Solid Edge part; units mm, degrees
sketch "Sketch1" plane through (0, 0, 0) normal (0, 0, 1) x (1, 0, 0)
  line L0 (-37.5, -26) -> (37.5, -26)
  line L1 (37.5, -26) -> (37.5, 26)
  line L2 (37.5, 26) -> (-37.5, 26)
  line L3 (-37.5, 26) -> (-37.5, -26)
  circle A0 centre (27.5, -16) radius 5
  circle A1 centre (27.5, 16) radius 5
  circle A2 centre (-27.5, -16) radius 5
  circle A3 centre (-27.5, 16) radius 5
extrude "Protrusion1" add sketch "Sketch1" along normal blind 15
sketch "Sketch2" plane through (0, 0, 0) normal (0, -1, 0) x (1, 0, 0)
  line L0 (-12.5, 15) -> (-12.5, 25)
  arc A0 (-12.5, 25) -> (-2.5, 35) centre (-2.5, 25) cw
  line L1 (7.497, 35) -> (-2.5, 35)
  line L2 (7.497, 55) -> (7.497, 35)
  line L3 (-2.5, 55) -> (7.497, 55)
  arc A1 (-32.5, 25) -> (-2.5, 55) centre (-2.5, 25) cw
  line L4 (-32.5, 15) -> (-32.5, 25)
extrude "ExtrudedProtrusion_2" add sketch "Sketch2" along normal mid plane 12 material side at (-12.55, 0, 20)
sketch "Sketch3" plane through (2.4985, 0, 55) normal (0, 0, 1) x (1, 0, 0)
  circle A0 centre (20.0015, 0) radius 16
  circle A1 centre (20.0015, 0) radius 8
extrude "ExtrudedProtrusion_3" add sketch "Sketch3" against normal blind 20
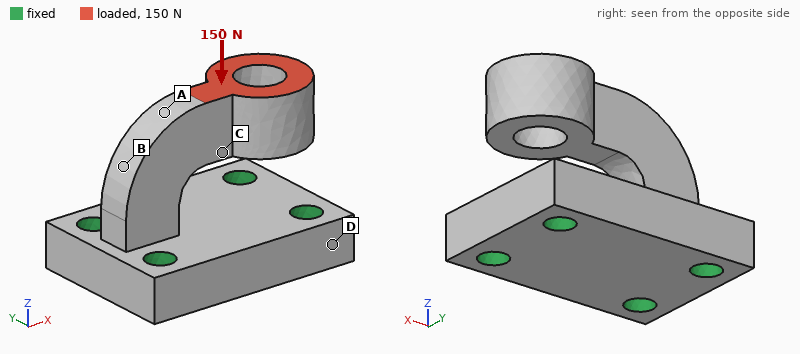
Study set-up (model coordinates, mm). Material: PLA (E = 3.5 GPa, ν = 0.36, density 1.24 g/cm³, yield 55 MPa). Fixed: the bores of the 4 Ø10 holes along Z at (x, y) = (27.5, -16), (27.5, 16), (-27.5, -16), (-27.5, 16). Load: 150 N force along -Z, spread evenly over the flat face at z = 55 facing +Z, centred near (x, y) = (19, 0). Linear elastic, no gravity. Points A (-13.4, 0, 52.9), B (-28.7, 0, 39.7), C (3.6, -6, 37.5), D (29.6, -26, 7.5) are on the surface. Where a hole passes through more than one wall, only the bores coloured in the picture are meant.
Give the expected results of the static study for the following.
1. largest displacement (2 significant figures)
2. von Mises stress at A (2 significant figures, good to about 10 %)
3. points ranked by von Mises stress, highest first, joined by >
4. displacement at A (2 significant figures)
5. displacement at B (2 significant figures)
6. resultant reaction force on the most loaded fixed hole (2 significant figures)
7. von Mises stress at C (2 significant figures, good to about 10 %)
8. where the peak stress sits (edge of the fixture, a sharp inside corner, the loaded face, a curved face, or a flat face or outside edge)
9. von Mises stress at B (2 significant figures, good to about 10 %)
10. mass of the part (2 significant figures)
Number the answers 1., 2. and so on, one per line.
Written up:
1. 0.66 mm
2. 3.9 MPa
3. B > A > C > D
4. 0.23 mm
5. 0.11 mm
6. 43 N
7. 2.5 MPa
8. a curved face
9. 4.9 MPa
10. 97 g
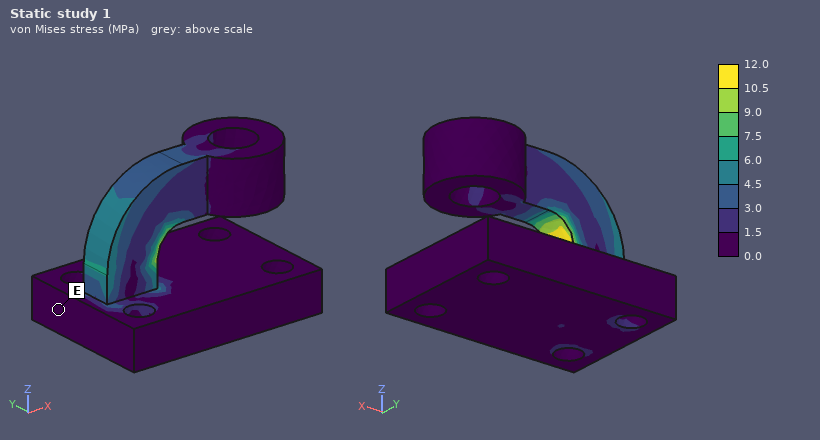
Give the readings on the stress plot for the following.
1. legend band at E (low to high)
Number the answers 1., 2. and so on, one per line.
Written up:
1. 0.0 to 1.5 MPa
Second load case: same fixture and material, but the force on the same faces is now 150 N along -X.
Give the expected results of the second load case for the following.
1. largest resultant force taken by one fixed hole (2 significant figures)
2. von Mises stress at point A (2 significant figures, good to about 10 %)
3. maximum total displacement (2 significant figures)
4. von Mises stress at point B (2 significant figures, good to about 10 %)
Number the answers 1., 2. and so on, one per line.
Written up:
1. 73 N
2. 2.1 MPa
3. 0.47 mm
4. 3.0 MPa
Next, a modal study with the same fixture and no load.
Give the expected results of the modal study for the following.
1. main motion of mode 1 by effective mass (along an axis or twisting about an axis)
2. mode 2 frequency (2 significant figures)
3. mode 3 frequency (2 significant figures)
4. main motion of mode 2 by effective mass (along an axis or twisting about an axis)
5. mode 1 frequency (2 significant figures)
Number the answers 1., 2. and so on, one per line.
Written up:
1. along Y
2. 630 Hz
3. 1300 Hz
4. along Z
5. 410 Hz
